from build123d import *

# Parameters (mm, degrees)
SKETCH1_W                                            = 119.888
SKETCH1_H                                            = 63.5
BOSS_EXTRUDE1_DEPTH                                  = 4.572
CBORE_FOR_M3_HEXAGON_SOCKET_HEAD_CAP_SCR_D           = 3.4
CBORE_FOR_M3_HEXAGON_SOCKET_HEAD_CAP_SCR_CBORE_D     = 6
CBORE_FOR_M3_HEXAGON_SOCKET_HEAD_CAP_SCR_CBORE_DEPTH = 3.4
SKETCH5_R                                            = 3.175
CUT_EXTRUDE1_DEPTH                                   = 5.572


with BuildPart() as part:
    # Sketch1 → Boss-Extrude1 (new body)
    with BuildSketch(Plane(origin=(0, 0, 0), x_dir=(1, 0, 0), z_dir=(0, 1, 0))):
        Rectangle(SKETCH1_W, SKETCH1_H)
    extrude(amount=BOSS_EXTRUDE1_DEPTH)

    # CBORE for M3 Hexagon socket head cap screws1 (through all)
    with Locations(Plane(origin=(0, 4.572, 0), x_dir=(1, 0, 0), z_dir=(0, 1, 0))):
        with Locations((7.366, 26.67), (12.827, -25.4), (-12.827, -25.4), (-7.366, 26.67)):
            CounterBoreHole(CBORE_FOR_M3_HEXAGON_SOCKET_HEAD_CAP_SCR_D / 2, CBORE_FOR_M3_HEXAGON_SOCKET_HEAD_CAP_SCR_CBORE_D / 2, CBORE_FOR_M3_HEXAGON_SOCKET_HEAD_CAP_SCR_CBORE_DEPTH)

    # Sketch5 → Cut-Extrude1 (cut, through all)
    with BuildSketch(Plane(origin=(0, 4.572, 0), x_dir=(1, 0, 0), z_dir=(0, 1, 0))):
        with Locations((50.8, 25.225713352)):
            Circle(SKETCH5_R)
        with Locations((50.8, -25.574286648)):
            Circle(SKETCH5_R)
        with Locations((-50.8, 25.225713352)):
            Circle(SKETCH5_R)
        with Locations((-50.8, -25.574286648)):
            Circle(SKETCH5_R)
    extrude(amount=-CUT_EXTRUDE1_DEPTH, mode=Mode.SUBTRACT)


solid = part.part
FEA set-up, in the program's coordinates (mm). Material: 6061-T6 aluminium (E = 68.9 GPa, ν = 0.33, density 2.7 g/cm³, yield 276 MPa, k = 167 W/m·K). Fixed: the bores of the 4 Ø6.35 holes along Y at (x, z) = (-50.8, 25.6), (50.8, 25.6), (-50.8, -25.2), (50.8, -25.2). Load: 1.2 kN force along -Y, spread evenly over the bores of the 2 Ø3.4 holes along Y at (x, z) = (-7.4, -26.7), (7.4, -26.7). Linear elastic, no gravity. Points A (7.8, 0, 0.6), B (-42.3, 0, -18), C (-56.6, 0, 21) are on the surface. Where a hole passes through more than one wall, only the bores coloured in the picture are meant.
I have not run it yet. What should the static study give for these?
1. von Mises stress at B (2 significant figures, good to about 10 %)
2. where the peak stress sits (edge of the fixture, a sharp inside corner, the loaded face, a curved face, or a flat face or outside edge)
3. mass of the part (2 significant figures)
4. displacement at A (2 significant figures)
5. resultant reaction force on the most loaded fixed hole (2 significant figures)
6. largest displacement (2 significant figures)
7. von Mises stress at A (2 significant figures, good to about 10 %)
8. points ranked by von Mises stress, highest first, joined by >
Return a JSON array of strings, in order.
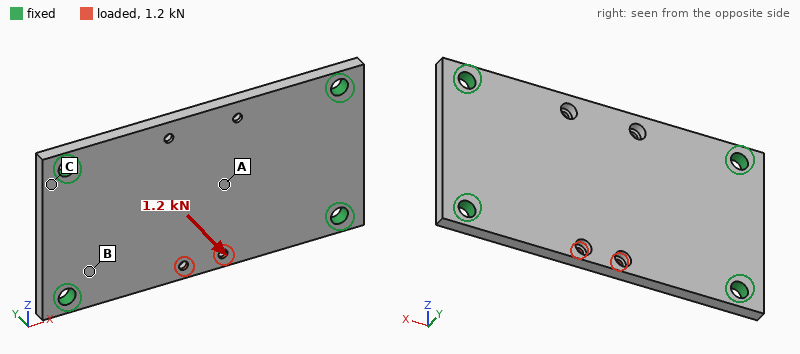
["75 MPa", "the loaded face", "91 g", "0.17 mm", "630 N", "0.47 mm", "46 MPa", "B > A > C"]
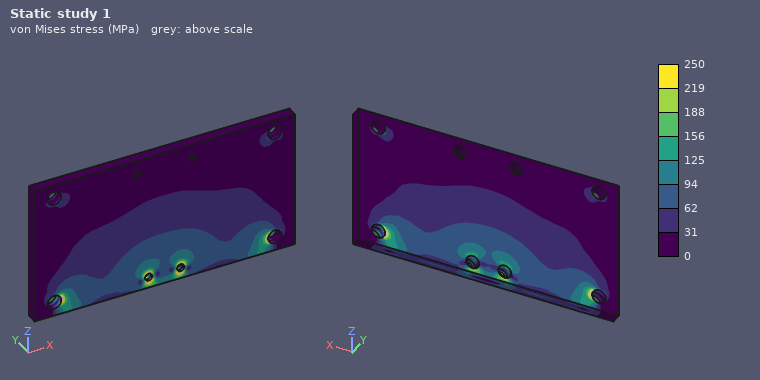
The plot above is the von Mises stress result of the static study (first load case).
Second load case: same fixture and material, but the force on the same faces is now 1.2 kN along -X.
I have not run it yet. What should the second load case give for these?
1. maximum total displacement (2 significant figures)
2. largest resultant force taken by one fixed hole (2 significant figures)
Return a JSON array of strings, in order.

["8.9 µm", "420 N"]
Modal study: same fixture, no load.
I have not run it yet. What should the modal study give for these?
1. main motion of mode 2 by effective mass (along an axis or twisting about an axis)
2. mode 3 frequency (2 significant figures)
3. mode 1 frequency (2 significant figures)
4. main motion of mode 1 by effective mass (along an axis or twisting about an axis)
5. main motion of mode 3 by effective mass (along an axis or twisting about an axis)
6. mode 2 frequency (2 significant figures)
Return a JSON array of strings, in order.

["twisting about X", "5800 Hz", "2200 Hz", "along Y", "twisting about Z", "3500 Hz"]
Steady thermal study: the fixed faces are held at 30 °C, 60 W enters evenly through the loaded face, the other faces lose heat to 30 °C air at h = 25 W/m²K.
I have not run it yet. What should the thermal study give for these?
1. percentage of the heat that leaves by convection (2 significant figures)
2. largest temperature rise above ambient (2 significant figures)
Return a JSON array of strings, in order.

["11 %", "76 K"]
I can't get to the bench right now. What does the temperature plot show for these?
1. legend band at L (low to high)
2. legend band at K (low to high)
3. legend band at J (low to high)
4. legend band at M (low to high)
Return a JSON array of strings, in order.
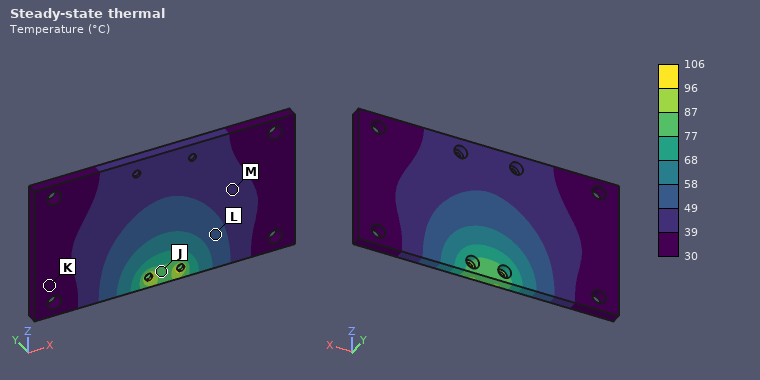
["49 to 58 °C", "30 to 39 °C", "77 to 87 °C", "39 to 49 °C"]
